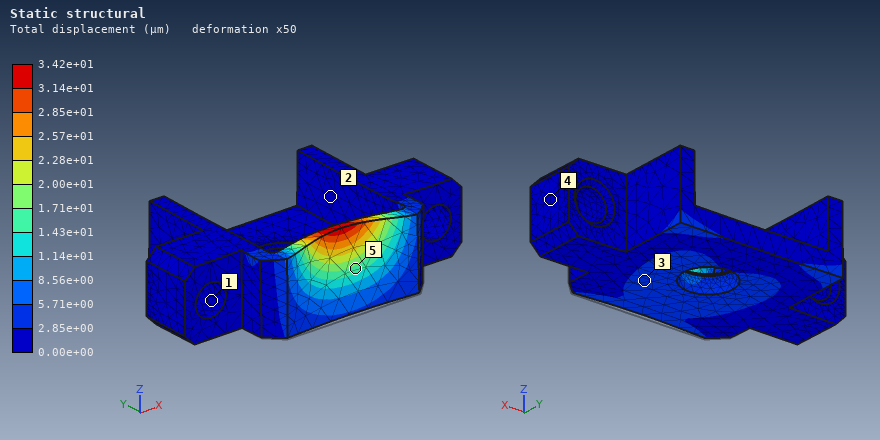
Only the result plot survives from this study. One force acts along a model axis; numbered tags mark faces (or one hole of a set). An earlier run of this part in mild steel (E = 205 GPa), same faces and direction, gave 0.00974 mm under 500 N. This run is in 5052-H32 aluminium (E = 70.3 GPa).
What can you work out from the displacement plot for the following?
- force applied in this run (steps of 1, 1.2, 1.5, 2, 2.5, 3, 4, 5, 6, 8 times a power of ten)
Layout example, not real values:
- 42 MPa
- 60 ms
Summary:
- 600 N
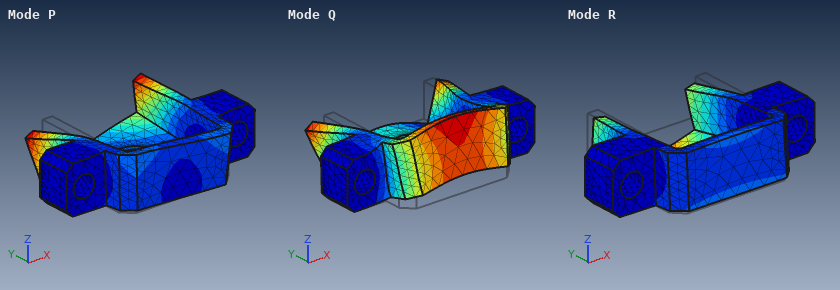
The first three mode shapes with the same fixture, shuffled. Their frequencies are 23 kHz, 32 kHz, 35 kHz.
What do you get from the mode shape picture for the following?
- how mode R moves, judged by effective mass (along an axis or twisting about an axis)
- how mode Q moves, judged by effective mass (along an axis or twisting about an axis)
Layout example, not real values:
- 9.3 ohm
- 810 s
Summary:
- along Z
- along Z
